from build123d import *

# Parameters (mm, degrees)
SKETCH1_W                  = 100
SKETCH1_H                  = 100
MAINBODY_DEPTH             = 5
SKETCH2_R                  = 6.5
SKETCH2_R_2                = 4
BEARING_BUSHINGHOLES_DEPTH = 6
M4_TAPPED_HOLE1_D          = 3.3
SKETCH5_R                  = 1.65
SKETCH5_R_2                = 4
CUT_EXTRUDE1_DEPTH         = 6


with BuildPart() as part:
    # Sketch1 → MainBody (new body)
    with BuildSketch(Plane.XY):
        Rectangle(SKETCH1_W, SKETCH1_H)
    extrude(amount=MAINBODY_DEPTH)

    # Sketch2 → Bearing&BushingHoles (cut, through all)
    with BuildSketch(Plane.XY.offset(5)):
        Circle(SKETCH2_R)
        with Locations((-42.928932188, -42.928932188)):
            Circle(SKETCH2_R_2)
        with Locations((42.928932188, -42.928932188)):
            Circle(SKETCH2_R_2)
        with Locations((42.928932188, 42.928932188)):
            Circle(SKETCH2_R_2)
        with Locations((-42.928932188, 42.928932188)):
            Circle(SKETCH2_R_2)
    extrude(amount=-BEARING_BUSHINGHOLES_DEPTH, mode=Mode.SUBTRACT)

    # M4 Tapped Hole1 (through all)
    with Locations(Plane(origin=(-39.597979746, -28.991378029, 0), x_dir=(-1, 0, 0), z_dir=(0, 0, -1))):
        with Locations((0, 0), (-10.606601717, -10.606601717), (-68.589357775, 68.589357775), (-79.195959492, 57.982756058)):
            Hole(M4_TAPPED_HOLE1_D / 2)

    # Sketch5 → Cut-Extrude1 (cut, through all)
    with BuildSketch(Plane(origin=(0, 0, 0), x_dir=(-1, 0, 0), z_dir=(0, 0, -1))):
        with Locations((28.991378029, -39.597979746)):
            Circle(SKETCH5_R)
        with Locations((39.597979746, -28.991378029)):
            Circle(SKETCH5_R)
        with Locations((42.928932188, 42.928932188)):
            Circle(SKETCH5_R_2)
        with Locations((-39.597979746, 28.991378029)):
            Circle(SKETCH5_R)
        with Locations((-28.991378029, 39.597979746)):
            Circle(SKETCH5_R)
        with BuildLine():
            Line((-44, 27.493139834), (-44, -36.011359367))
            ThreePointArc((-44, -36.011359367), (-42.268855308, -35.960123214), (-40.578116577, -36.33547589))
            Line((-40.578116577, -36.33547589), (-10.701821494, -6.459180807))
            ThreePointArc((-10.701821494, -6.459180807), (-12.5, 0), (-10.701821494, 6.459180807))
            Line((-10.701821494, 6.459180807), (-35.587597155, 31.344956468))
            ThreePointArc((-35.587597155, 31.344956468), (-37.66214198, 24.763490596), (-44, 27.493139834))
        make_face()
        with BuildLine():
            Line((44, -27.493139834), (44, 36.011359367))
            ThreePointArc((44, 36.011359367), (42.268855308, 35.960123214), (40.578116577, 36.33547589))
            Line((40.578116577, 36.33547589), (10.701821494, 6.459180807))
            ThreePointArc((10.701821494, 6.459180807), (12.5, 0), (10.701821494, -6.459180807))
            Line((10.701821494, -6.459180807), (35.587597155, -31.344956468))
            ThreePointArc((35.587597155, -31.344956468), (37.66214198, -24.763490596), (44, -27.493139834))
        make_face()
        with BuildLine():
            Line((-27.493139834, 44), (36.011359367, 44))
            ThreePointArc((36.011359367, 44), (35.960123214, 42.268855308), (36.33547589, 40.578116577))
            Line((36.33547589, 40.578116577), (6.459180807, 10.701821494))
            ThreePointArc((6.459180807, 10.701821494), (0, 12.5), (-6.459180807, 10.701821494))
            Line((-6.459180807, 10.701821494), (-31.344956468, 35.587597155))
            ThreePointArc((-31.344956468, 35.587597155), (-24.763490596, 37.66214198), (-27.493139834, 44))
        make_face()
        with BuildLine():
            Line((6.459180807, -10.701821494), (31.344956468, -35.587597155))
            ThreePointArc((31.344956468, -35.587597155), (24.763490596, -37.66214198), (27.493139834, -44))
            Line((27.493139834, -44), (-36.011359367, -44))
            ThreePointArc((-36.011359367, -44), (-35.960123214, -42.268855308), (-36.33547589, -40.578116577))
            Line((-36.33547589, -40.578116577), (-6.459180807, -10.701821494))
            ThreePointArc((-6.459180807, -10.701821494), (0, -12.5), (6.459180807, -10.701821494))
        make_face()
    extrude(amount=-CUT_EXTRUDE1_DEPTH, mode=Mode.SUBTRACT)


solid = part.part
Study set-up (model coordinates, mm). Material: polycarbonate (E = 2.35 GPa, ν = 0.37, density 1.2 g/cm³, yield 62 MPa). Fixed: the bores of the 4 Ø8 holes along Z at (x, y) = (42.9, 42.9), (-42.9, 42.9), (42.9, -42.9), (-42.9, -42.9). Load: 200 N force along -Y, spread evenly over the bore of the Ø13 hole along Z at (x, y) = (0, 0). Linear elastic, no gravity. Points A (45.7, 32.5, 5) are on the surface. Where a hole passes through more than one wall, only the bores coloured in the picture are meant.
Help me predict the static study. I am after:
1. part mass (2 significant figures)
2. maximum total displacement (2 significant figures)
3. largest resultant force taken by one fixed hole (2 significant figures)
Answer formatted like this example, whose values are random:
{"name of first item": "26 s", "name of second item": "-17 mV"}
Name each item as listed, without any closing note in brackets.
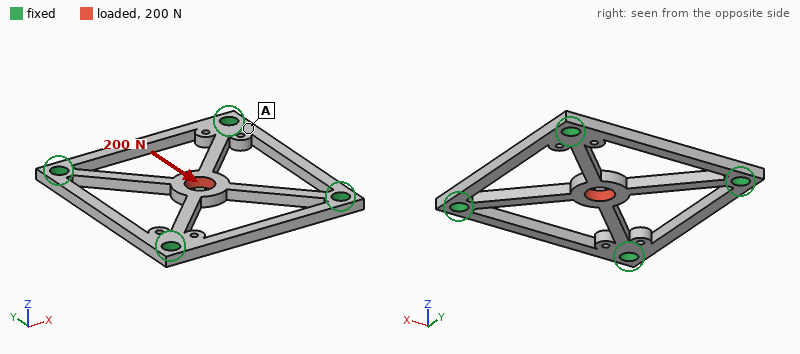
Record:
{"part mass": "24 g", "maximum total displacement": "75 µm", "largest resultant force taken by one fixed hole": "69 N"}
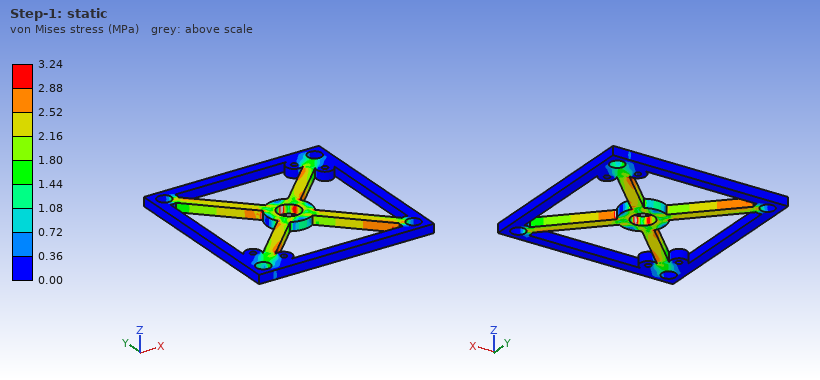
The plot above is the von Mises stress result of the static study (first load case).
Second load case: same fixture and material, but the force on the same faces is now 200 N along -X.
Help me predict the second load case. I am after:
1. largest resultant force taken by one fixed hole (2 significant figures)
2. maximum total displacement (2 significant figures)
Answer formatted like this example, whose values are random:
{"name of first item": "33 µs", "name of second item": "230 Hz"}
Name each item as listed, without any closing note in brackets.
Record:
{"largest resultant force taken by one fixed hole": "69 N", "maximum total displacement": "75 µm"}
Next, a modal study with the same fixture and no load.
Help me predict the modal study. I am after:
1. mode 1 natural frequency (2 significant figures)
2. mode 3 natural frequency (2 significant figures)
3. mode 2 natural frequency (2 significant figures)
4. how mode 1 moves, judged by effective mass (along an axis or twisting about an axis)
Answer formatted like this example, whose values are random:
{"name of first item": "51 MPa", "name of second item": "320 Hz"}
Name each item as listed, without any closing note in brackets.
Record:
{"mode 1 natural frequency": "610 Hz", "mode 3 natural frequency": "1200 Hz", "mode 2 natural frequency": "1200 Hz", "how mode 1 moves, judged by effective mass": "along Z"}
